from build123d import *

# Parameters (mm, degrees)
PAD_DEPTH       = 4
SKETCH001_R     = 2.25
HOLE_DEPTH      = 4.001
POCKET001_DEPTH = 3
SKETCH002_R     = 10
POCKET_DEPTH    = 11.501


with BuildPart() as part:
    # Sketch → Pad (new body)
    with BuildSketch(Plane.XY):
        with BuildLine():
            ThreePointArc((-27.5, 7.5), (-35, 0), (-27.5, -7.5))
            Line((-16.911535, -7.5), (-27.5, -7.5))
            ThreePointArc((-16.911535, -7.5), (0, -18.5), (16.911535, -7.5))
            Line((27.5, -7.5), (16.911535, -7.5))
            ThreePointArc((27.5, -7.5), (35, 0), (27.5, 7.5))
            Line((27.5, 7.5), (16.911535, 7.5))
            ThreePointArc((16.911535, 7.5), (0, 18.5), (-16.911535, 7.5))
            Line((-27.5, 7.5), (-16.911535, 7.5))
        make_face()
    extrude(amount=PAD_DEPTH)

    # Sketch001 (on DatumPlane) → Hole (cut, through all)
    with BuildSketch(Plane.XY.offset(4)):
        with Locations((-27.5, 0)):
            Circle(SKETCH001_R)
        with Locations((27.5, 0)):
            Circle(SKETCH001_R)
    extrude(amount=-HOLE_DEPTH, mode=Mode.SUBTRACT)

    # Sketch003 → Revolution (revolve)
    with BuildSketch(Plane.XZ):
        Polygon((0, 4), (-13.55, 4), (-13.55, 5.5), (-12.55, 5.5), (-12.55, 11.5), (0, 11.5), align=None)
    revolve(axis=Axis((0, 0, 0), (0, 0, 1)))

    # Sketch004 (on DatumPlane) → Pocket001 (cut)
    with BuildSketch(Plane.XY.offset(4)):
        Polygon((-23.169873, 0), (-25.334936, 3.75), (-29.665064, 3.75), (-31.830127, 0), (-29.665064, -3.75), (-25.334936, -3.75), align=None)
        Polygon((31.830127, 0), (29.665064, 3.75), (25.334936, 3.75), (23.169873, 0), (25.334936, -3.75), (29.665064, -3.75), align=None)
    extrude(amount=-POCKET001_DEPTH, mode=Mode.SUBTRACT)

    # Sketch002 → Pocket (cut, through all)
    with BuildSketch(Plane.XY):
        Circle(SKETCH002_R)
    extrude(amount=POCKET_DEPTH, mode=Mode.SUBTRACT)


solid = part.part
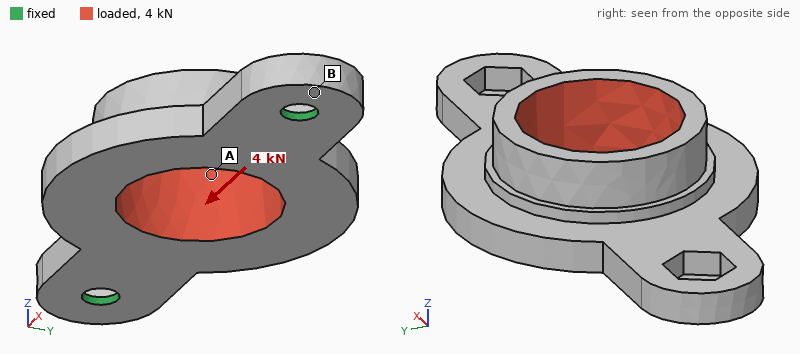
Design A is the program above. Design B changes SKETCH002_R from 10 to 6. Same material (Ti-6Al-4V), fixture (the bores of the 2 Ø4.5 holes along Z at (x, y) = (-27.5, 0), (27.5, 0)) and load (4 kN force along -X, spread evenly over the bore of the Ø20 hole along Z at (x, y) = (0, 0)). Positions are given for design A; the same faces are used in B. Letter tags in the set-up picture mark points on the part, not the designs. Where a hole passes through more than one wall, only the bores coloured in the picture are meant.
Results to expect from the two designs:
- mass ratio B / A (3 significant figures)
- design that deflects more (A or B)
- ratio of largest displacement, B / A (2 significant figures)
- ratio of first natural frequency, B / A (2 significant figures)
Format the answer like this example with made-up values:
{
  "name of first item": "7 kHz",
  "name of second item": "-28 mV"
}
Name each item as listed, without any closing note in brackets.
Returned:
{
  "mass ratio B / A": "1.38",
  "design that deflects more": "A",
  "ratio of largest displacement, B / A": "0.83",
  "ratio of first natural frequency, B / A": "0.89"
}
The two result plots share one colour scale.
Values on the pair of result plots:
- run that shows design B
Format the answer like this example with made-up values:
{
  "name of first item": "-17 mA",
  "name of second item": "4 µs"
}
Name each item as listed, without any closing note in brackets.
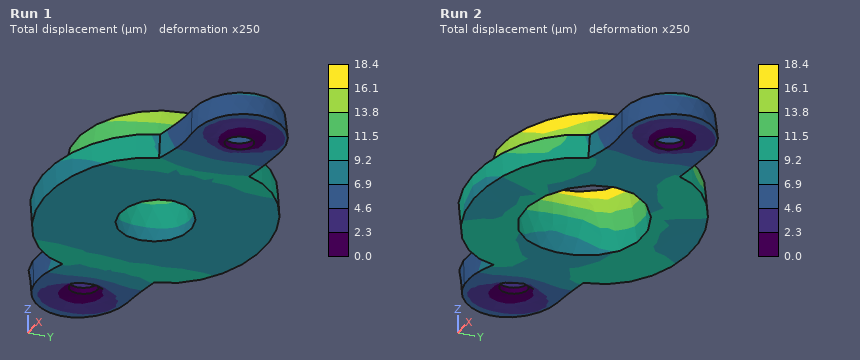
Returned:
{
  "run that shows design B": "Run 1"
}
